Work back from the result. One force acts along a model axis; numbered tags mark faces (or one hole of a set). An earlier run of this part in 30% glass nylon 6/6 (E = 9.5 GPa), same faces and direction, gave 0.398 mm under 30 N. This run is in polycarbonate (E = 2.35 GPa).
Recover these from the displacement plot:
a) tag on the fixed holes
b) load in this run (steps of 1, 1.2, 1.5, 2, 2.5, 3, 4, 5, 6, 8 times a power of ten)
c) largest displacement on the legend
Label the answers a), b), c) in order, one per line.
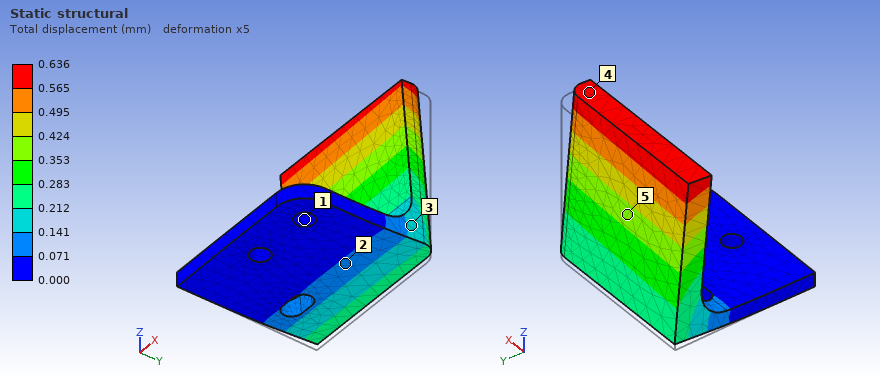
a) 1
b) 12 N
c) 0.636 mm
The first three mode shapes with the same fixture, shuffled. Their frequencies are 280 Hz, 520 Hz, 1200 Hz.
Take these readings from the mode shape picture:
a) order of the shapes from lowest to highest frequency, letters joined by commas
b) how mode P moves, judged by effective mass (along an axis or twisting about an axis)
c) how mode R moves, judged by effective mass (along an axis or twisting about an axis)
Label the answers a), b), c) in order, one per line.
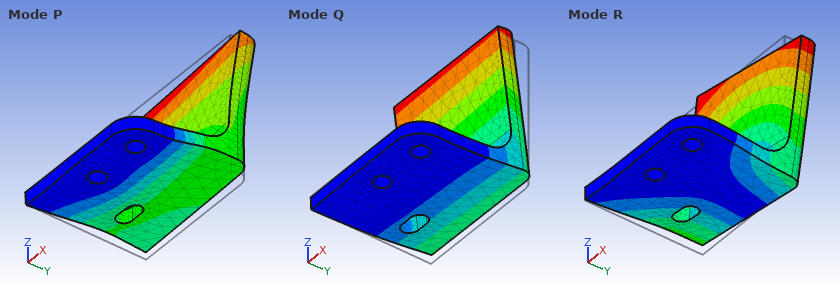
a) Q, R, P
b) along Z
c) along X
